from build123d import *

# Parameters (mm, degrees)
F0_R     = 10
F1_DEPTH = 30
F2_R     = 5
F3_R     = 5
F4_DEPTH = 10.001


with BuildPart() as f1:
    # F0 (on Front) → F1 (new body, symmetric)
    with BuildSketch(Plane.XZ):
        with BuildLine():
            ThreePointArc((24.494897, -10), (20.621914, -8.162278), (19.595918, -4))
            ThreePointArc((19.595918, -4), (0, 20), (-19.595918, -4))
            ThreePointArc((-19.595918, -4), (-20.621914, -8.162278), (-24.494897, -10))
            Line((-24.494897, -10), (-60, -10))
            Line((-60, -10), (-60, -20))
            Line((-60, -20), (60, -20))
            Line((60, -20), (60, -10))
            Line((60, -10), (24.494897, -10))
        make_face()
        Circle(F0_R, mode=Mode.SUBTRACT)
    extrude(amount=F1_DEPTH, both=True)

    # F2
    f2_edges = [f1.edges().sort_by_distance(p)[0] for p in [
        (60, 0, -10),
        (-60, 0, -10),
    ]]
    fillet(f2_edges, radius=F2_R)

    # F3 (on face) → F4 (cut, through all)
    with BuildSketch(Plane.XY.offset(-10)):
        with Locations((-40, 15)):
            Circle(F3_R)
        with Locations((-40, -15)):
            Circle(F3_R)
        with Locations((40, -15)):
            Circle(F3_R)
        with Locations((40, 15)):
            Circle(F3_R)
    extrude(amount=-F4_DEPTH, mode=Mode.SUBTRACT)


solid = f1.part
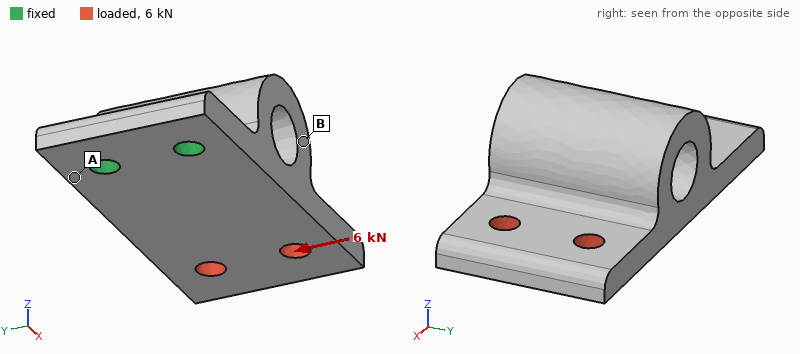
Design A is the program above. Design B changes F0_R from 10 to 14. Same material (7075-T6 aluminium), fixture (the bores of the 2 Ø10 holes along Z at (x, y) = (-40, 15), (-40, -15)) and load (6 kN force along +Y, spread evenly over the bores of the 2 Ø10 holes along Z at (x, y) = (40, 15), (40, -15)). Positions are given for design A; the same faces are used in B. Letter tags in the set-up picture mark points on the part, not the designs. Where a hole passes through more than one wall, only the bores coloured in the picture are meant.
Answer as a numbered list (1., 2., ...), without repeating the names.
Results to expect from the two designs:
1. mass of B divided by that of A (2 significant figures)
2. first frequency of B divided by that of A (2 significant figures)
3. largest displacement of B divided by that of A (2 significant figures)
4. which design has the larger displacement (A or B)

1. 0.84
2. 0.97
3. 1.2
4. B
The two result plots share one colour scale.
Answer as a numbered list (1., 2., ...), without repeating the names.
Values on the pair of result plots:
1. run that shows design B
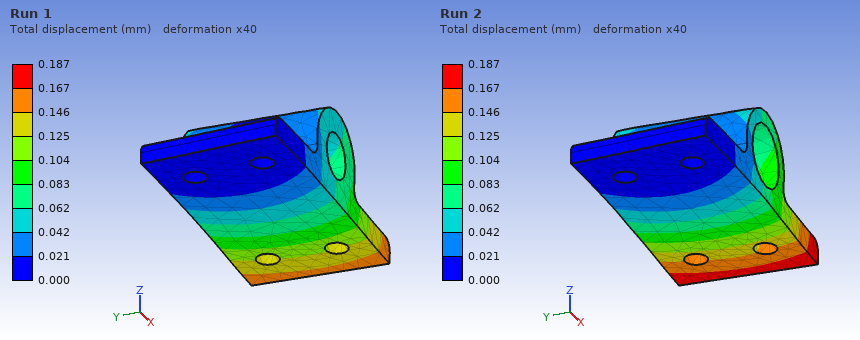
1. Run 2
